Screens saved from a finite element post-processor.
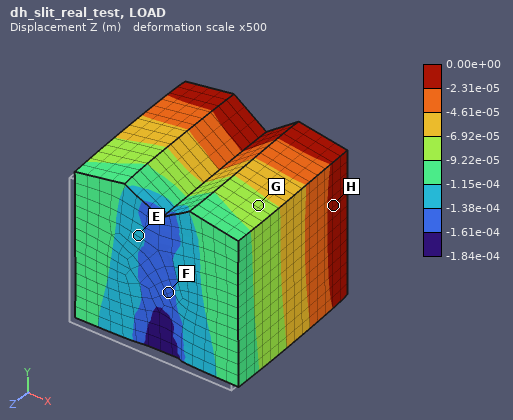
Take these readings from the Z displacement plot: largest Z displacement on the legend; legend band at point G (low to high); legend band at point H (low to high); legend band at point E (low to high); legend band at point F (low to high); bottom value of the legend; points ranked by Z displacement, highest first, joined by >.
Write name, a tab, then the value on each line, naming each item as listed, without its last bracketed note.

largest Z displacement on the legend	0.00e+00 m
legend band at point G	-9.22e-05 to -6.92e-05 m
legend band at point H	-2.31e-05 to 0.00e+00 m
legend band at point E	-1.38e-04 to -1.15e-04 m
legend band at point F	-1.61e-04 to -1.38e-04 m
bottom value of the legend	-1.84e-04 m
points ranked by Z displacement, highest first, joined by >	H > G > E > F
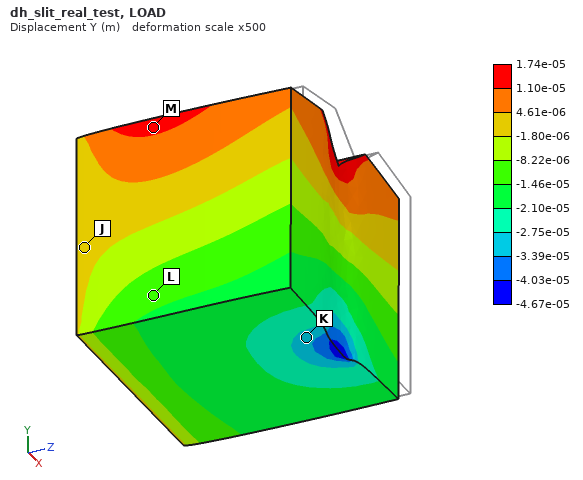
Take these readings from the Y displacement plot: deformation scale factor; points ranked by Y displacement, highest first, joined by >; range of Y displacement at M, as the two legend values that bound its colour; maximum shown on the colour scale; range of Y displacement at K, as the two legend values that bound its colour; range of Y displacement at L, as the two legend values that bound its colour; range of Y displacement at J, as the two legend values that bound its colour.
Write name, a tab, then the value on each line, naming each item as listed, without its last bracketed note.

deformation scale factor	500
points ranked by Y displacement, highest first, joined by >	M > J > L > K
range of Y displacement at M, as the two legend values that bound its colour	1.10e-05 to 1.74e-05 m
maximum shown on the colour scale	1.74e-05 m
range of Y displacement at K, as the two legend values that bound its colour	-3.39e-05 to -2.75e-05 m
range of Y displacement at L, as the two legend values that bound its colour	-1.46e-05 to -8.22e-06 m
range of Y displacement at J, as the two legend values that bound its colour	-1.80e-06 to 4.61e-06 m
